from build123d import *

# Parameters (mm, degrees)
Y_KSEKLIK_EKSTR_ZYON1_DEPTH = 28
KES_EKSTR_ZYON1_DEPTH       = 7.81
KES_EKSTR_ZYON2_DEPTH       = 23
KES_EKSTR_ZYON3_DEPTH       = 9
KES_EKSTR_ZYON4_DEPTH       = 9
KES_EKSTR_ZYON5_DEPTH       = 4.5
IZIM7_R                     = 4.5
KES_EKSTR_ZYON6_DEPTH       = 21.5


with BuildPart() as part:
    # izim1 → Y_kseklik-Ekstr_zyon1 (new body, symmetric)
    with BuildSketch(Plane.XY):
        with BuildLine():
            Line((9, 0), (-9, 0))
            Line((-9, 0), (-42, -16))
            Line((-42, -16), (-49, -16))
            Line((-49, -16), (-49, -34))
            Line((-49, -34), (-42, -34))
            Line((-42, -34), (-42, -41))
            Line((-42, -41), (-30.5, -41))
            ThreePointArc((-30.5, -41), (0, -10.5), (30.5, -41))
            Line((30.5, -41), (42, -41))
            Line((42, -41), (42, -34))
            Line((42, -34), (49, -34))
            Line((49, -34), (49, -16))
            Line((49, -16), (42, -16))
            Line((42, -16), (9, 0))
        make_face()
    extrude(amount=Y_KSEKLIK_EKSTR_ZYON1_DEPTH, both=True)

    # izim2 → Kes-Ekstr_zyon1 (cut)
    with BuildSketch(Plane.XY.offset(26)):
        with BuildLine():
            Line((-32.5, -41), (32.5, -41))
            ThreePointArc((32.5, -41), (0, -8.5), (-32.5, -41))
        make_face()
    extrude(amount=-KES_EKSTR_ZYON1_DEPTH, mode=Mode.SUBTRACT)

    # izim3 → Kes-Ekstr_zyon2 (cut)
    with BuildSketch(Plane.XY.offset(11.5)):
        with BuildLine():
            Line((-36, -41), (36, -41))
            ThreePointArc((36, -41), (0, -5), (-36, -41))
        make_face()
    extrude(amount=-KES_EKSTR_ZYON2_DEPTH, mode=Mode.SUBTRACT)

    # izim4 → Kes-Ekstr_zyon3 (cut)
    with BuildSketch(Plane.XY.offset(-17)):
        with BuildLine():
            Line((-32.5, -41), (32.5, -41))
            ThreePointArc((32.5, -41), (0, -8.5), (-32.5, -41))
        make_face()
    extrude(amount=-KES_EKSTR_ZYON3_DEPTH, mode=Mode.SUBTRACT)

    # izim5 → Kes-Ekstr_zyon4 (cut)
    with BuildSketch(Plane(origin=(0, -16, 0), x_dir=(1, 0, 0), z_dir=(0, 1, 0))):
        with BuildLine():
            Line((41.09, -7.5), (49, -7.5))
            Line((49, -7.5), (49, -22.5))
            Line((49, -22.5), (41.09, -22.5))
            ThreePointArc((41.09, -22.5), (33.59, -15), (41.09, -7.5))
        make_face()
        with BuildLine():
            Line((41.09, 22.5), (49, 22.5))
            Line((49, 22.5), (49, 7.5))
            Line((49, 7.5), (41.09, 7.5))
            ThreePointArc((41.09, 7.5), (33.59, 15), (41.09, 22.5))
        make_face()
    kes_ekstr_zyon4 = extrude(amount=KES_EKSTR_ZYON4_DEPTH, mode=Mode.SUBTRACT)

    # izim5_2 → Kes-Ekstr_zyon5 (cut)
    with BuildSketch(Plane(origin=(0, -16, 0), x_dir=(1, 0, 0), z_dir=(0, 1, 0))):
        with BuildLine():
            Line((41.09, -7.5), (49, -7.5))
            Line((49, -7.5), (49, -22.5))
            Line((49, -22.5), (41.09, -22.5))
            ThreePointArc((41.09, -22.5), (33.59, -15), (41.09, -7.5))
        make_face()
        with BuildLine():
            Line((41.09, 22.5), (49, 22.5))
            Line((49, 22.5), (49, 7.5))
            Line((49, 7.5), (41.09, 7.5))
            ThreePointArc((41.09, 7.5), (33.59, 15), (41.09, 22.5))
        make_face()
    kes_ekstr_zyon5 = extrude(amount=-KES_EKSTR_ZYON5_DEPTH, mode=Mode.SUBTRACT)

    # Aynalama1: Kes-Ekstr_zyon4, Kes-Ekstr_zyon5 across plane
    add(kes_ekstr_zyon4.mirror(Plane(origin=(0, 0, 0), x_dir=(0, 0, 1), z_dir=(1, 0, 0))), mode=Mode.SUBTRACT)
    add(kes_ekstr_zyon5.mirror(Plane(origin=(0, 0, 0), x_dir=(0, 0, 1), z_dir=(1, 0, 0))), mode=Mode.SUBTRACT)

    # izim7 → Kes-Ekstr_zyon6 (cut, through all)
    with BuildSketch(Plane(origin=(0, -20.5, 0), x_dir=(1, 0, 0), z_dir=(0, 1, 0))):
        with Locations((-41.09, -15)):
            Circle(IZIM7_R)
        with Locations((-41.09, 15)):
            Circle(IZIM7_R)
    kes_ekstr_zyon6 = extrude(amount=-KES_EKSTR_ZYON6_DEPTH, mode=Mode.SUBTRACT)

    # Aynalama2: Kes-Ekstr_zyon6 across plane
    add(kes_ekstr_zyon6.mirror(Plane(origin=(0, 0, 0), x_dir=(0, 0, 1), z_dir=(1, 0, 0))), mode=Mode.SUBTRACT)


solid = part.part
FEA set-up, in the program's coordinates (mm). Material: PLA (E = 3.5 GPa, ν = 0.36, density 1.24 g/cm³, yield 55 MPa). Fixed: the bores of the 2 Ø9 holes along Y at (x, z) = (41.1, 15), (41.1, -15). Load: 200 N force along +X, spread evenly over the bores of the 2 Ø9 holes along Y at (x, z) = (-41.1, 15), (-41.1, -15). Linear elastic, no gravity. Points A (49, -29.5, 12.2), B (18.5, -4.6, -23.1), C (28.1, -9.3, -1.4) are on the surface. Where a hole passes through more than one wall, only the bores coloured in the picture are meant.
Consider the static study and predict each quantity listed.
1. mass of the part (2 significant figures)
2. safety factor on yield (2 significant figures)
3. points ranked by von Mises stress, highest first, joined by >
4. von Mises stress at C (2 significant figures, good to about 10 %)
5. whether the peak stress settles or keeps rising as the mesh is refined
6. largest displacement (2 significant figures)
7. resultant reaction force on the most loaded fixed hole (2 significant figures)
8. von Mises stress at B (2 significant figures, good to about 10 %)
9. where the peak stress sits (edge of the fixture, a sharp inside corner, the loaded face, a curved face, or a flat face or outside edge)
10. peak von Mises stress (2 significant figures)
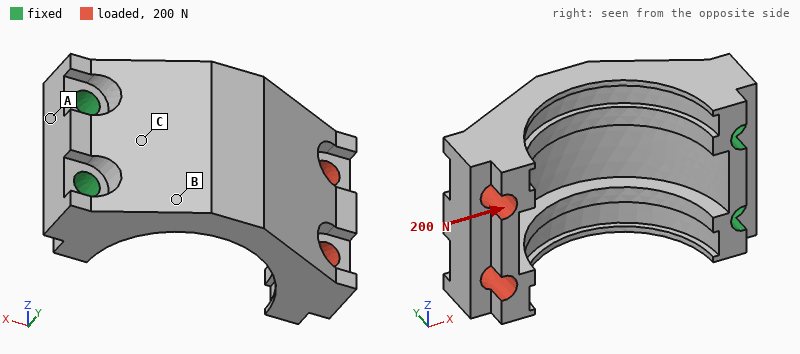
87 g
4.5
B > C > A
2.6 MPa
settles
1.3 mm
100 N
5.7 MPa
a curved face
12 MPa
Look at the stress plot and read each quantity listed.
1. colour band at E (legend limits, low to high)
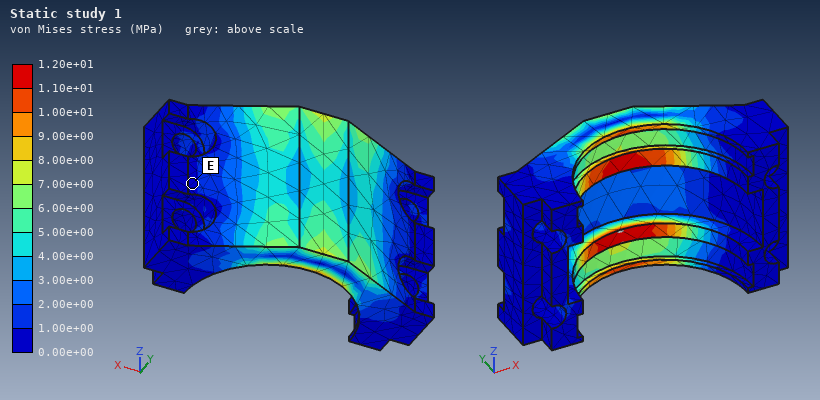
0.00e+00 to 1.00e+00 MPa
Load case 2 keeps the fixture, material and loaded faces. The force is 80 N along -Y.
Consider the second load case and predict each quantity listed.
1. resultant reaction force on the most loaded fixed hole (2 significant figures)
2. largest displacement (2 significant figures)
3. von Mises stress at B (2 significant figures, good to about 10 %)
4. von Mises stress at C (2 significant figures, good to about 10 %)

43 N
1.2 mm
6.5 MPa
4.8 MPa
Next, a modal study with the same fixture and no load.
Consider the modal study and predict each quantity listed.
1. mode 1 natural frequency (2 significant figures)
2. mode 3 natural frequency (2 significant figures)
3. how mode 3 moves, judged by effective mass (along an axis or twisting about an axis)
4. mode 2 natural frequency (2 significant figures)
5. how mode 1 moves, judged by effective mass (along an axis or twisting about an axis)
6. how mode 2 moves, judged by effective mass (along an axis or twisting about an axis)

260 Hz
980 Hz
along X
420 Hz
along Y
along Z
